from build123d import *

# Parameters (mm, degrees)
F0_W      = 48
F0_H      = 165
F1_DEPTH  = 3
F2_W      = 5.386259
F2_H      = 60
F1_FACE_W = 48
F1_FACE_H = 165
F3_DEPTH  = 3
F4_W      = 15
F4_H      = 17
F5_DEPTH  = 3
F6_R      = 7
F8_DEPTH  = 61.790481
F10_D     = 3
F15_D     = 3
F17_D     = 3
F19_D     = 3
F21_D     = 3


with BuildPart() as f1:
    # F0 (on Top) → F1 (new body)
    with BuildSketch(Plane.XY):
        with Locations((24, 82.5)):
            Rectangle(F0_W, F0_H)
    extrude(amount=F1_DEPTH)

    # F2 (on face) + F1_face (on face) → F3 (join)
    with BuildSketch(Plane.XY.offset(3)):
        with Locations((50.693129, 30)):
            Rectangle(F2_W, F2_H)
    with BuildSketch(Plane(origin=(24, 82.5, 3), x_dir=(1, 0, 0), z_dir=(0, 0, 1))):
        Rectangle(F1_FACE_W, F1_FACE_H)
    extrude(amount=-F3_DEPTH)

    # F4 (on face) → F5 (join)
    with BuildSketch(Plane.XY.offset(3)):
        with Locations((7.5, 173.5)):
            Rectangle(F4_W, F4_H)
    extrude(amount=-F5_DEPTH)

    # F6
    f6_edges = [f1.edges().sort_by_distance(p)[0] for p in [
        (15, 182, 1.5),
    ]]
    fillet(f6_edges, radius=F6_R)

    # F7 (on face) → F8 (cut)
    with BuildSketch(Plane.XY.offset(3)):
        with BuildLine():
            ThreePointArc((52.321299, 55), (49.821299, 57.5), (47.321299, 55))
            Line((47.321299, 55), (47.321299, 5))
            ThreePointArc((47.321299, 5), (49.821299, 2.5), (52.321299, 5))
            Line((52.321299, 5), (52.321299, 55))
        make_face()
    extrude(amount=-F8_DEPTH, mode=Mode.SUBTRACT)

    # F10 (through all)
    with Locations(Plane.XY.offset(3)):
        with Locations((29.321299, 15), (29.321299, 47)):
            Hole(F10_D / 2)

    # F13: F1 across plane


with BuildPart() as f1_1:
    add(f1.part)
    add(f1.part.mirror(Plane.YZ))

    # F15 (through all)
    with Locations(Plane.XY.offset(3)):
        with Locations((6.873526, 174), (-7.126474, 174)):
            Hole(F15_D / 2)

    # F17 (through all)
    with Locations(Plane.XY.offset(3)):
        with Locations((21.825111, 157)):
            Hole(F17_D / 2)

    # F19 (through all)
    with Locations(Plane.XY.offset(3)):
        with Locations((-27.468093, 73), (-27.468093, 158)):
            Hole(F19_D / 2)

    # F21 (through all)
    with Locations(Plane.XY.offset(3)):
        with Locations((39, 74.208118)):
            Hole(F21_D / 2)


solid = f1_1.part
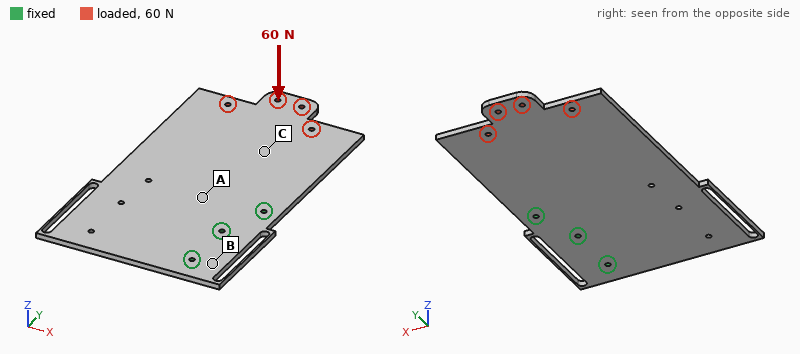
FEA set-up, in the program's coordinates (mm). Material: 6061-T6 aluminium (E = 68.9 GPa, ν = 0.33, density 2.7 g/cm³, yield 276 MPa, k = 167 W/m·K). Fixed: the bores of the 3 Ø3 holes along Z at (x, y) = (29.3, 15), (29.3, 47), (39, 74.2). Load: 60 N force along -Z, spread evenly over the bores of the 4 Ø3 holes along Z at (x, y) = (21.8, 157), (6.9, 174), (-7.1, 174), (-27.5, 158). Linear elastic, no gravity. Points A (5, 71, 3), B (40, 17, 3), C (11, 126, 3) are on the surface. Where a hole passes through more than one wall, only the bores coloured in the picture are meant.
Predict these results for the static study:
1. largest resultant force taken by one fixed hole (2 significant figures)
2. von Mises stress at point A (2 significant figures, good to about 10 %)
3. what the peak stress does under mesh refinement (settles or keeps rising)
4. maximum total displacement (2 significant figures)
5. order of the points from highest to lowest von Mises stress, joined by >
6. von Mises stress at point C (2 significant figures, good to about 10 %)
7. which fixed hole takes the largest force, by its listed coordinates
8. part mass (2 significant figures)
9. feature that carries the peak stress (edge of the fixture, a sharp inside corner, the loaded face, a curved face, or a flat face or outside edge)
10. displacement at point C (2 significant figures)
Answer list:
130 N
29 MPa
keeps rising
2.3 mm
A > C > B
17 MPa
(39, 74.2)
130 g
edge of the fixture
0.83 mm
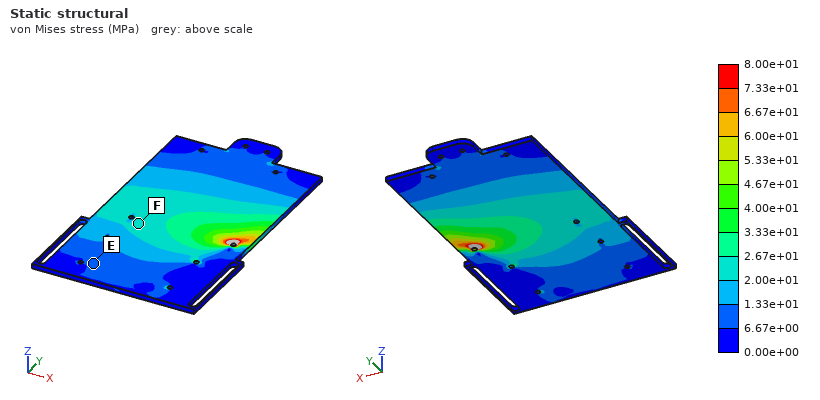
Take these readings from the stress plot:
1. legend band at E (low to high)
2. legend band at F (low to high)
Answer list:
6.67e+00 to 1.33e+01 MPa
2.00e+01 to 2.67e+01 MPa
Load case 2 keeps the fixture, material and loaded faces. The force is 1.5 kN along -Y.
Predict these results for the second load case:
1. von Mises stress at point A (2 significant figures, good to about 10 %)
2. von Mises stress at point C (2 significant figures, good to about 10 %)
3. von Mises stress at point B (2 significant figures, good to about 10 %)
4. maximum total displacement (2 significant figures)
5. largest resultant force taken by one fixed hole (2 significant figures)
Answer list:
9.0 MPa
6.5 MPa
4.8 MPa
44 µm
970 N
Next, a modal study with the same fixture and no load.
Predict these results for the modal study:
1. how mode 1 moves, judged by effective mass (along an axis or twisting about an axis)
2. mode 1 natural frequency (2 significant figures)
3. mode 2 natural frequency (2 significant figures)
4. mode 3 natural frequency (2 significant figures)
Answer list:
along Z
180 Hz
350 Hz
620 Hz
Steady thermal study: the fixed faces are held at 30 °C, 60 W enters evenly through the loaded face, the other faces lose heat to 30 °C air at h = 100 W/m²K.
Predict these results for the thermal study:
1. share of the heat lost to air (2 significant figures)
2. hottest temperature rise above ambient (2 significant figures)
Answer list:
88 %
77 K
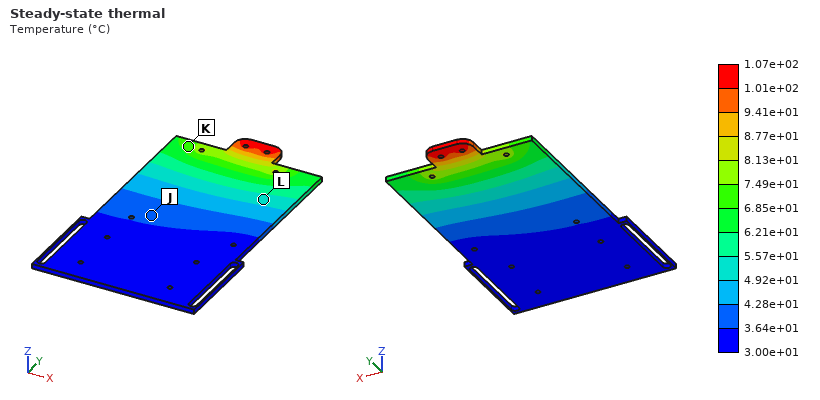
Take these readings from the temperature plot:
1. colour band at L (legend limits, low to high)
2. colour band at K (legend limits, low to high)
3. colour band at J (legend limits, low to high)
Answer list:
4.92e+01 to 5.57e+01 °C
6.85e+01 to 7.49e+01 °C
3.64e+01 to 4.28e+01 °C
